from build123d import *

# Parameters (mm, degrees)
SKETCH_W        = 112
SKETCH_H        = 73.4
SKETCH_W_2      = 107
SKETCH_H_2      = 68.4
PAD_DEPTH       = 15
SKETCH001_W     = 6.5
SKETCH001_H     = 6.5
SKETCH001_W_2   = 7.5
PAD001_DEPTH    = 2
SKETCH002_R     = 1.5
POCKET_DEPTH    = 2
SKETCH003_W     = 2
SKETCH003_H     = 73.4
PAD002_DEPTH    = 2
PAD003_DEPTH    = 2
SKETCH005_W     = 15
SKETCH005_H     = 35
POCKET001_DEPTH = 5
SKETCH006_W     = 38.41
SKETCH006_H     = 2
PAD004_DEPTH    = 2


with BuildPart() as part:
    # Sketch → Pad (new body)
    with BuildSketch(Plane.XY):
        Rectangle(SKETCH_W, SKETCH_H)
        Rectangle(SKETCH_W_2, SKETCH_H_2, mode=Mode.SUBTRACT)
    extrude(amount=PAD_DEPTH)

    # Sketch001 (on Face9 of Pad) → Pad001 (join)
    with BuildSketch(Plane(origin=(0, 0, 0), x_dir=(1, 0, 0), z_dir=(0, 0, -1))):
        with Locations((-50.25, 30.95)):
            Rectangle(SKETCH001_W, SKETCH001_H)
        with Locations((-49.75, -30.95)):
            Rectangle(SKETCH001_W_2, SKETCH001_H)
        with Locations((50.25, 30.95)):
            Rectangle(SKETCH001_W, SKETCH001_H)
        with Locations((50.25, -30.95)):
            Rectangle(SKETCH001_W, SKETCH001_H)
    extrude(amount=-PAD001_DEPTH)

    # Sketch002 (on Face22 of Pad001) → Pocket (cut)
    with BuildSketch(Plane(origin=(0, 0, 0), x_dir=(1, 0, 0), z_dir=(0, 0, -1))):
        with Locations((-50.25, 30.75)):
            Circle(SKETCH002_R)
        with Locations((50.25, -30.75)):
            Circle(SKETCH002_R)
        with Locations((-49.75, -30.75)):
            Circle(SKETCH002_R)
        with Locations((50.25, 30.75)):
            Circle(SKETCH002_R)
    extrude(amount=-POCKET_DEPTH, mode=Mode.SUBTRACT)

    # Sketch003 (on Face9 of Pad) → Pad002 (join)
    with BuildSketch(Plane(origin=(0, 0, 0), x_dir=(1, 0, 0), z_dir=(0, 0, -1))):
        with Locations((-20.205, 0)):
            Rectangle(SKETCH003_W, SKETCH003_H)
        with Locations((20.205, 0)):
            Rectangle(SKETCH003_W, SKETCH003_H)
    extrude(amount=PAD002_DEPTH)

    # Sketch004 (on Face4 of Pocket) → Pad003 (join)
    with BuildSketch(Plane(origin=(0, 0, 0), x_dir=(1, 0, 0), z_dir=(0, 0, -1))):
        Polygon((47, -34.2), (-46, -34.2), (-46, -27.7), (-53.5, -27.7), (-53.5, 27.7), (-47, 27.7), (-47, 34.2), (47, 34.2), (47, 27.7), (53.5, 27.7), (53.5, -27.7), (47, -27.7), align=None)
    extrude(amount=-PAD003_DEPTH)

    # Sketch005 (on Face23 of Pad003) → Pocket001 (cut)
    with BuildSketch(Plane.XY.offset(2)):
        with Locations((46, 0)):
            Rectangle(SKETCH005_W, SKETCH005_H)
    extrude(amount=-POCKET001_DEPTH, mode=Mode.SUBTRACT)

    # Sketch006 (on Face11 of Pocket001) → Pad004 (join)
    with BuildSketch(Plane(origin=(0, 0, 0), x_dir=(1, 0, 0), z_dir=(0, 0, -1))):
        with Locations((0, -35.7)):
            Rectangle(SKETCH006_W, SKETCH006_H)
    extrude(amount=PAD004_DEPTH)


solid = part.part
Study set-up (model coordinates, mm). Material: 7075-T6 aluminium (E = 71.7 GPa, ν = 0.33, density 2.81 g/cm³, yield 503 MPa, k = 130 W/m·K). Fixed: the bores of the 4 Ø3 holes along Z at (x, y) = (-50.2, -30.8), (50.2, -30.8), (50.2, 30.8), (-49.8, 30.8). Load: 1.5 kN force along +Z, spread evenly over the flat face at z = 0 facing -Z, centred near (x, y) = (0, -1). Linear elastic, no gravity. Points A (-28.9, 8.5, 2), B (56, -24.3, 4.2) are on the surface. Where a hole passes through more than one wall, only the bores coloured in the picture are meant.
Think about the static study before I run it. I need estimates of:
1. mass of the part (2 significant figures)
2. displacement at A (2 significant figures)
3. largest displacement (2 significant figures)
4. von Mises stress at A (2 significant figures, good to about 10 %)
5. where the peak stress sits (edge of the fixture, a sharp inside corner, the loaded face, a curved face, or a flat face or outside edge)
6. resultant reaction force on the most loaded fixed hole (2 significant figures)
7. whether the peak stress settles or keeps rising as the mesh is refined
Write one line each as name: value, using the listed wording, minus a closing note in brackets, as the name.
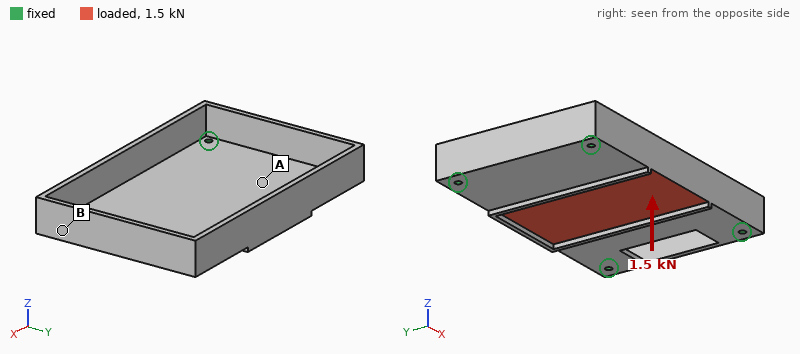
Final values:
mass of the part: 78 g
displacement at A: 0.34 mm
largest displacement: 0.74 mm
von Mises stress at A: 53 MPa
where the peak stress sits: edge of the fixture
resultant reaction force on the most loaded fixed hole: 700 N
whether the peak stress settles or keeps rising as the mesh is refined: keeps rising
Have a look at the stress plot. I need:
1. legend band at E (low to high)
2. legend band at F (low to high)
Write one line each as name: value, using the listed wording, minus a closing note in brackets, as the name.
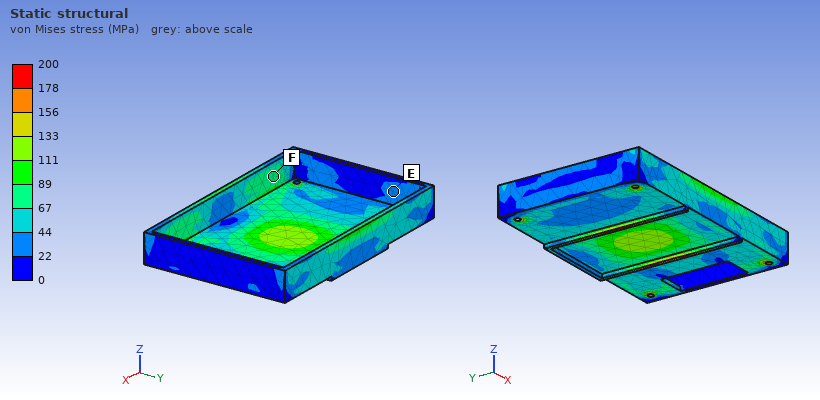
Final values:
legend band at E: 22 to 44 MPa
legend band at F: 67 to 89 MPa
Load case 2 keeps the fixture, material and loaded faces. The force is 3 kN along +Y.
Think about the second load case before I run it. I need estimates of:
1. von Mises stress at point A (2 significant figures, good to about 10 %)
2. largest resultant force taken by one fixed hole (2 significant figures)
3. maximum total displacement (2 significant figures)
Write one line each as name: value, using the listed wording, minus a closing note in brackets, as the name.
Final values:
von Mises stress at point A: 26 MPa
largest resultant force taken by one fixed hole: 1.1 kN
maximum total displacement: 37 µm
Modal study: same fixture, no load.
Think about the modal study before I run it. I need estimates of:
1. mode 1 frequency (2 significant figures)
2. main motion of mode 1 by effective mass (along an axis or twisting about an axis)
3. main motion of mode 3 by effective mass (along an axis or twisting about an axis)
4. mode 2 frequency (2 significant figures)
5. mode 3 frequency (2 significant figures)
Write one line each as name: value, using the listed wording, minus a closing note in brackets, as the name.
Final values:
mode 1 frequency: 1700 Hz
main motion of mode 1 by effective mass: along Z
main motion of mode 3 by effective mass: twisting about X
mode 2 frequency: 3000 Hz
mode 3 frequency: 3700 Hz
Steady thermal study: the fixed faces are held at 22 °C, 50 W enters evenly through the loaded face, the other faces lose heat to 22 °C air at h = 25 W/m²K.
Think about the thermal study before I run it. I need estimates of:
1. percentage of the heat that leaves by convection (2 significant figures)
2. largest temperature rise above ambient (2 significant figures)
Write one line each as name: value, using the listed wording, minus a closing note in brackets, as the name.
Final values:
percentage of the heat that leaves by convection: 27 %
largest temperature rise above ambient: 49 K
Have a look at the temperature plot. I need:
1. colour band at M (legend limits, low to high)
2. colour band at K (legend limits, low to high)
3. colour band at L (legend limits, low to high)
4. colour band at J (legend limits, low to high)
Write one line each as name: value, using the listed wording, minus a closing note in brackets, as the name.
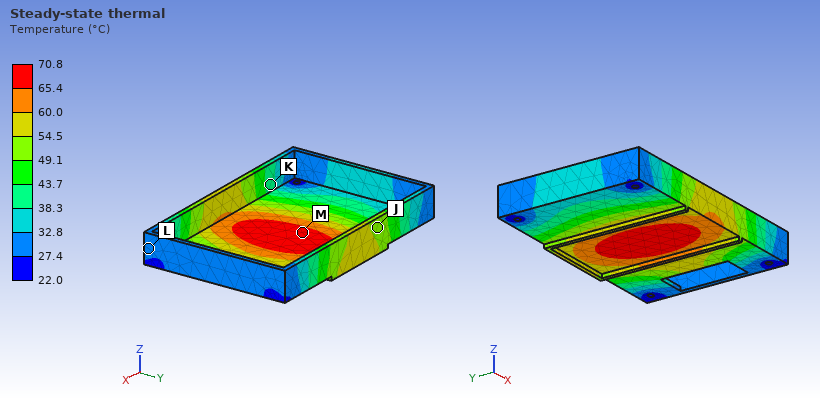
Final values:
colour band at M: 65.4 to 70.8 °C
colour band at K: 38.3 to 43.7 °C
colour band at L: 27.4 to 32.8 °C
colour band at J: 49.1 to 54.5 °C
